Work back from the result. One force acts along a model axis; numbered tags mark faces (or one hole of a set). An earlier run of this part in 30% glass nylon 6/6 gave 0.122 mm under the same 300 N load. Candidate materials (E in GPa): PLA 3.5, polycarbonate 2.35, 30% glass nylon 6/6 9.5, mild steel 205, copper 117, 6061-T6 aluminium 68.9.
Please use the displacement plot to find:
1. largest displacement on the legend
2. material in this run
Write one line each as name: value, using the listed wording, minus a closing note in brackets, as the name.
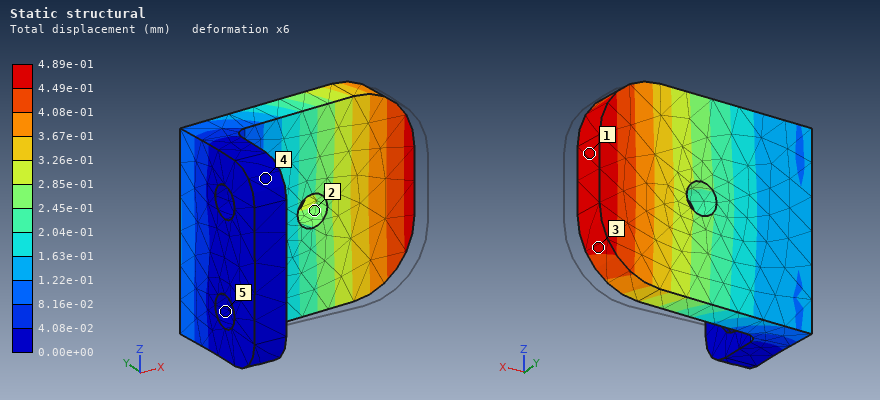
largest displacement on the legend: 4.89e-01 mm
material in this run: polycarbonate
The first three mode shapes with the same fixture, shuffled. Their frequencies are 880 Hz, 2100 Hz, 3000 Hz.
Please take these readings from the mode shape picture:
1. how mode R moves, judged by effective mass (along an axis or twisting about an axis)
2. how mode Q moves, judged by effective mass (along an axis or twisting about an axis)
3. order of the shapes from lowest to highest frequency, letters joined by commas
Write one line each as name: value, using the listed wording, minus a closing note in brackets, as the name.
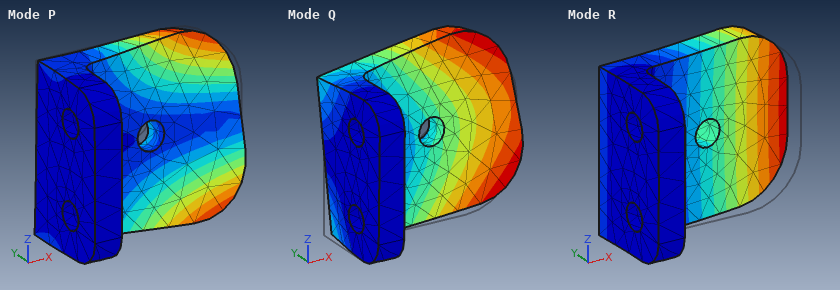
how mode R moves, judged by effective mass: along Y
how mode Q moves, judged by effective mass: along Z
order of the shapes from lowest to highest frequency, letters joined by commas: R, Q, P
